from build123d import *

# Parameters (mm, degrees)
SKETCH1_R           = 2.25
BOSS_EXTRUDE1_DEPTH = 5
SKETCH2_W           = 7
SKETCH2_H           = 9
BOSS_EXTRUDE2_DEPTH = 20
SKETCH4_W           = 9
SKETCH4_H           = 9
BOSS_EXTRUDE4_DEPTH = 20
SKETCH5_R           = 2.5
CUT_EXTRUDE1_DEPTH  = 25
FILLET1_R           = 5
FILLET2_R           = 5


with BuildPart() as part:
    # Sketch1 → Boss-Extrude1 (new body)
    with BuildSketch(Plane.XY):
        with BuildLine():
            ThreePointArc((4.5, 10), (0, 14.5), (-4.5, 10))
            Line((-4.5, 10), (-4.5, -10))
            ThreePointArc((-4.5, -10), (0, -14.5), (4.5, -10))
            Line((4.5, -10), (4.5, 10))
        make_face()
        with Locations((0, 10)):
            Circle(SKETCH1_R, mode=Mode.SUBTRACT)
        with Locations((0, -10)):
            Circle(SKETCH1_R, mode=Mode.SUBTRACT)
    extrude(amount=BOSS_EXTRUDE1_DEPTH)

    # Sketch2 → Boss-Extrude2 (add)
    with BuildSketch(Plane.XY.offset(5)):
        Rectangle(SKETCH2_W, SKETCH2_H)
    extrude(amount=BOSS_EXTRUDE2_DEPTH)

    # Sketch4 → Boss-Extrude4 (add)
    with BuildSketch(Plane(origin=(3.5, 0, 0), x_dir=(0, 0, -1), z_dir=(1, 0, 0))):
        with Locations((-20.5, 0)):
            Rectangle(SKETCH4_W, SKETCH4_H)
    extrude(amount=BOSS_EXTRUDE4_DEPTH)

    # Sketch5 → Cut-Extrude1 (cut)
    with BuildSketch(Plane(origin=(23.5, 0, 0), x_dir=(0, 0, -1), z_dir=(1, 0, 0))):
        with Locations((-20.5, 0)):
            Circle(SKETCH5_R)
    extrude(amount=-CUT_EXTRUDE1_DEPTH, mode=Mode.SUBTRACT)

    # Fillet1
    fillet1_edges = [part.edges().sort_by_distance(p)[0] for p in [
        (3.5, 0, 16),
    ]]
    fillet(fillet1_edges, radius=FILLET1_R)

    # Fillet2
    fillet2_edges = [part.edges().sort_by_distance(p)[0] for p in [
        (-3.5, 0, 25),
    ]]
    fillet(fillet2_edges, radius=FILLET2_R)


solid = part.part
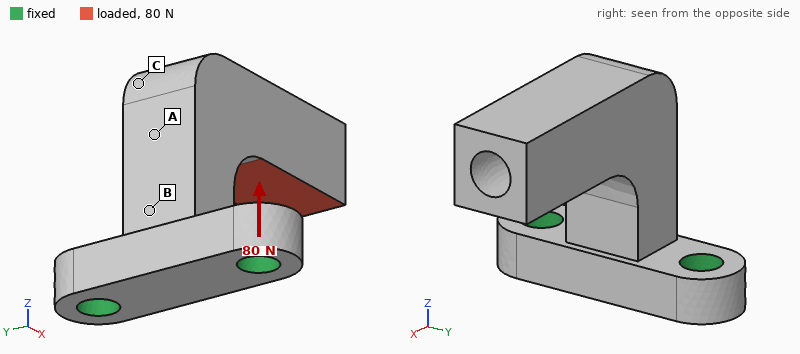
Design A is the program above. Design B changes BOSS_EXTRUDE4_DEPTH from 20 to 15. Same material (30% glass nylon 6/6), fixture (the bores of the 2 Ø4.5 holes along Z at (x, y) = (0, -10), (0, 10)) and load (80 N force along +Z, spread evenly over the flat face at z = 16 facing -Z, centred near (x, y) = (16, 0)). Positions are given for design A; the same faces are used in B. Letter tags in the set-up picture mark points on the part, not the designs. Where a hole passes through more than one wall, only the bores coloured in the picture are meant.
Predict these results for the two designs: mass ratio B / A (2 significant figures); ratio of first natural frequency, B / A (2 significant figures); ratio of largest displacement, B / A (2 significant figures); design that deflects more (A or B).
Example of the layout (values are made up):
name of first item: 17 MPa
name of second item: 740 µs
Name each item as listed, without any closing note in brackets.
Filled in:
mass ratio B / A: 0.91
ratio of first natural frequency, B / A: 1.2
ratio of largest displacement, B / A: 0.71
design that deflects more: A
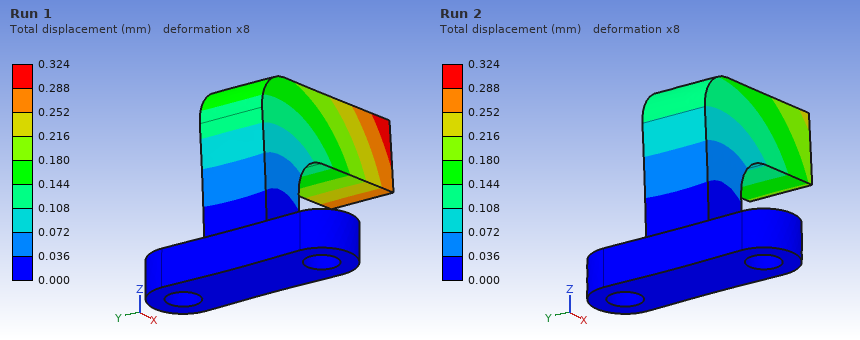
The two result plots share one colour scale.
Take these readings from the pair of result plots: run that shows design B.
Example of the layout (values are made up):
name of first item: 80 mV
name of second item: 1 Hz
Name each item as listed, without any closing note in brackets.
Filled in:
run that shows design B: Run 2
